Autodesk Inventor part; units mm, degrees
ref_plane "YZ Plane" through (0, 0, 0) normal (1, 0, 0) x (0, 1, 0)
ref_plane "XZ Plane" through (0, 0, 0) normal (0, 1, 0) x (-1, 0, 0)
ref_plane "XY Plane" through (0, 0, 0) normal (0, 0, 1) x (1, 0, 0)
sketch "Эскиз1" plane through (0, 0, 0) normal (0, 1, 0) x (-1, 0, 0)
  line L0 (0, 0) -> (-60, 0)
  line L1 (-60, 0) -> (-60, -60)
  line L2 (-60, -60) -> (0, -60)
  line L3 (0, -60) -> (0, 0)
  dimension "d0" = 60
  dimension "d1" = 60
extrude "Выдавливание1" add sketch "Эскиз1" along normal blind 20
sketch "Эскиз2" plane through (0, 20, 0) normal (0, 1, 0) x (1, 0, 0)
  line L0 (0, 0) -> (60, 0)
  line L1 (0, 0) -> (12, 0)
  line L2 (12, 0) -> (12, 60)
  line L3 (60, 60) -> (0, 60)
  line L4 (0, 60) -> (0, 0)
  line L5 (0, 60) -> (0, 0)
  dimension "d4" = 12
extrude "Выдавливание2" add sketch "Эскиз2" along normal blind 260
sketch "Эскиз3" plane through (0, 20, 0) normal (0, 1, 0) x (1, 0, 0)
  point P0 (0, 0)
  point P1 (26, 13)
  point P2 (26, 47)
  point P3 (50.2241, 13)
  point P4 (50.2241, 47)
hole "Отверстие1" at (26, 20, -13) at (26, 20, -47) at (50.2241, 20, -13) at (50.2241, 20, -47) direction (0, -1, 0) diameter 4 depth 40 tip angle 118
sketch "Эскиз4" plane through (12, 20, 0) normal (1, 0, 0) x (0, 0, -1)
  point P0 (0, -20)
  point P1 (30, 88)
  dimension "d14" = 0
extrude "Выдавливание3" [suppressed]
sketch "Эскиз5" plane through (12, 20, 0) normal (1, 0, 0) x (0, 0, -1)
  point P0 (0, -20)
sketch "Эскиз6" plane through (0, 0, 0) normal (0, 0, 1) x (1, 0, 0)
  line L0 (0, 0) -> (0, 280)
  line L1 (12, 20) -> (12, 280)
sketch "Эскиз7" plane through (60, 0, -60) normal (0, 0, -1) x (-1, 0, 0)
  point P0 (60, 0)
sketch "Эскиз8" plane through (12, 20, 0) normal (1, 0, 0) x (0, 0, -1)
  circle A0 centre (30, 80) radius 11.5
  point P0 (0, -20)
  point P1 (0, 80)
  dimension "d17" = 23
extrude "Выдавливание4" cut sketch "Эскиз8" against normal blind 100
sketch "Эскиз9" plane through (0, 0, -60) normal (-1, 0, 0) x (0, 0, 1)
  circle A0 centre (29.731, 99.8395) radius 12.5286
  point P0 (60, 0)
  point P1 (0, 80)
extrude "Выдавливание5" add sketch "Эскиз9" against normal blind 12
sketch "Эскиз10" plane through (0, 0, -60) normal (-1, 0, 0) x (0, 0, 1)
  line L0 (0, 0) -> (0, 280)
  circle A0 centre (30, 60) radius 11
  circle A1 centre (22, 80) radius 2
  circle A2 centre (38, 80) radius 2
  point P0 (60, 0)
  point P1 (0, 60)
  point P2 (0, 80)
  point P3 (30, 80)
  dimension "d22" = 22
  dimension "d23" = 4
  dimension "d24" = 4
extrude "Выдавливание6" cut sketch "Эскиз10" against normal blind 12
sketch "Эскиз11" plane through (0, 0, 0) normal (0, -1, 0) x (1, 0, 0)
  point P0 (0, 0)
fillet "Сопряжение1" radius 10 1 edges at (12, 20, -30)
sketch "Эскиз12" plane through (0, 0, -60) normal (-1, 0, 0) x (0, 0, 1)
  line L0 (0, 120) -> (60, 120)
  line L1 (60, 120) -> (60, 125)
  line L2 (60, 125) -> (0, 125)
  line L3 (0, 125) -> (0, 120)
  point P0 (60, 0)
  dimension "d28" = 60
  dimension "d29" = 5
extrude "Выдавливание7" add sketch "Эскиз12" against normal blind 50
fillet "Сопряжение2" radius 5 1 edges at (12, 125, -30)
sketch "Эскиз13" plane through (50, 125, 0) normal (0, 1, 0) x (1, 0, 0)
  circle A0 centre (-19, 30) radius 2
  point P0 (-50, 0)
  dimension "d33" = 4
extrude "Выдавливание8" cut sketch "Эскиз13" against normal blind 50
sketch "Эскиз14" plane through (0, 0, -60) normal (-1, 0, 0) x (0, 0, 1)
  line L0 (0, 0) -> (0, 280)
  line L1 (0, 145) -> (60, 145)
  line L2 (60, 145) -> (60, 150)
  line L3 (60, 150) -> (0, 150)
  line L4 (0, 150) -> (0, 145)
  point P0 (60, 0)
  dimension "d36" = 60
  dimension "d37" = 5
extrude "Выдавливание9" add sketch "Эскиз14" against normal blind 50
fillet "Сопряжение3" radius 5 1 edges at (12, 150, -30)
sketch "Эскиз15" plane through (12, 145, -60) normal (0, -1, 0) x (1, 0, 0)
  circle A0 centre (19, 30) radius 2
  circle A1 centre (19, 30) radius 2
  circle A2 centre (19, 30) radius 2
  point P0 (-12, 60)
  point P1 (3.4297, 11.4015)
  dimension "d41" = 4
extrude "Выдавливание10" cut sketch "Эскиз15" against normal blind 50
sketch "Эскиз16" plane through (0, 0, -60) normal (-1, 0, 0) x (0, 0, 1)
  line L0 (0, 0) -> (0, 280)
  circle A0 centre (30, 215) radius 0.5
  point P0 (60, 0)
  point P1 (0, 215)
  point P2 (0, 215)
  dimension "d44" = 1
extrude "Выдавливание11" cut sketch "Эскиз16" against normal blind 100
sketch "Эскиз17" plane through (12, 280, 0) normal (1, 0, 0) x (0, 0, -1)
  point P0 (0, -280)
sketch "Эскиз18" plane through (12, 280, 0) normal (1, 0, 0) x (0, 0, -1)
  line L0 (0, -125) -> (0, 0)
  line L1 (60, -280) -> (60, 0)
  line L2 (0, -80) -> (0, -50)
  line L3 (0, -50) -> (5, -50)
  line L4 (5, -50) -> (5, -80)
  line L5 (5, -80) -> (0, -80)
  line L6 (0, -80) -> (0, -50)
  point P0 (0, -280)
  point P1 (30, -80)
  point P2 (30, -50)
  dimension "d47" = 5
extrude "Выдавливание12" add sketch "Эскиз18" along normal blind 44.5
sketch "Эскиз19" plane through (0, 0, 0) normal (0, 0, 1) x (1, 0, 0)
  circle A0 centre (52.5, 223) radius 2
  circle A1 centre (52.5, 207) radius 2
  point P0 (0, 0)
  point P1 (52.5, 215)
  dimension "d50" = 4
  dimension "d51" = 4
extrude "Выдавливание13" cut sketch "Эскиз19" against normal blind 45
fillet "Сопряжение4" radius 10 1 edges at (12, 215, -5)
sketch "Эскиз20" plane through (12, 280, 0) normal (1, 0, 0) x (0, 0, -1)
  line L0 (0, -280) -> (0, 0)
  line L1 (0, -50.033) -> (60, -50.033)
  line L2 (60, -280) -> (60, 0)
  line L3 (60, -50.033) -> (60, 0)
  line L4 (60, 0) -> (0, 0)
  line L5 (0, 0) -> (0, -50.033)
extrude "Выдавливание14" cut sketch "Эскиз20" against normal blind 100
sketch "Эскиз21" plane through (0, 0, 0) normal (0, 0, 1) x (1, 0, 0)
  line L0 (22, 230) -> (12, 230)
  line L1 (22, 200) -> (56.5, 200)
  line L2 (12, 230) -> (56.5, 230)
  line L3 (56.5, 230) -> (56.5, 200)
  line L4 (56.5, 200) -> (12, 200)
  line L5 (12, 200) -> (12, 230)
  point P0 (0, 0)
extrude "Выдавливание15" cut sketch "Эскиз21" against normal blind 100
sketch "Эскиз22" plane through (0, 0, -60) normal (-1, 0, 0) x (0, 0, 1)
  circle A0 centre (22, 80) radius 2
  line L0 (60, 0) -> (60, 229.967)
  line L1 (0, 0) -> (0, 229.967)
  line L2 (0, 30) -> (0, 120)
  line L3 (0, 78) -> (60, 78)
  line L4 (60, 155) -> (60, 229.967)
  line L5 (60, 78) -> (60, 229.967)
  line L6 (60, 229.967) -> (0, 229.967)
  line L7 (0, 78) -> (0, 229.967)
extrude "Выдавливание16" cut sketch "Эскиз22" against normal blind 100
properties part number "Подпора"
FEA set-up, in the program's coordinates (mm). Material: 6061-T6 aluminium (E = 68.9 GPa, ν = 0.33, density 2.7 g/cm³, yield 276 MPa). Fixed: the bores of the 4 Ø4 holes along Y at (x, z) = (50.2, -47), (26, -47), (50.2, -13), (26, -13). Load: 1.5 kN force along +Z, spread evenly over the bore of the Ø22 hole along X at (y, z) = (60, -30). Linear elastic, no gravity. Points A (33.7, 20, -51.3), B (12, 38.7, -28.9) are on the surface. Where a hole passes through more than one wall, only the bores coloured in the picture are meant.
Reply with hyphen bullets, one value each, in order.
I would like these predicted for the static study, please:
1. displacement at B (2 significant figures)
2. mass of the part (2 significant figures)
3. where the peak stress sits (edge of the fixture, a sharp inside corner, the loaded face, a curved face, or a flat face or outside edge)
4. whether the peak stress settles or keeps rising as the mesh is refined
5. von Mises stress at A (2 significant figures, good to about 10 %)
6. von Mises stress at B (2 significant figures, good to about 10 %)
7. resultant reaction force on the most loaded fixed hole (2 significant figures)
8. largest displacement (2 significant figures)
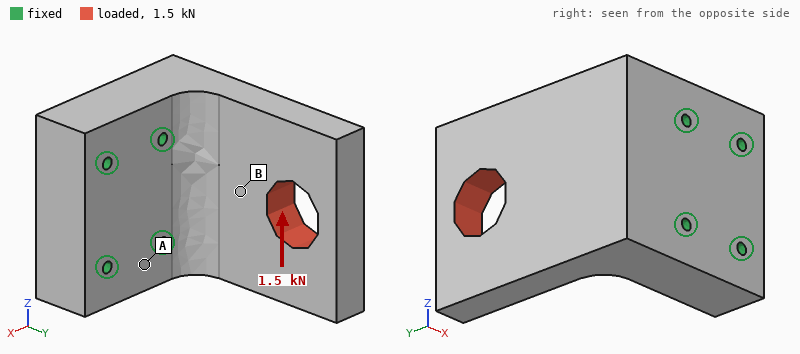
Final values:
- 11 µm
- 300 g
- edge of the fixture
- keeps rising
- 3.2 MPa
- 9.1 MPa
- 1.9 kN
- 31 µm
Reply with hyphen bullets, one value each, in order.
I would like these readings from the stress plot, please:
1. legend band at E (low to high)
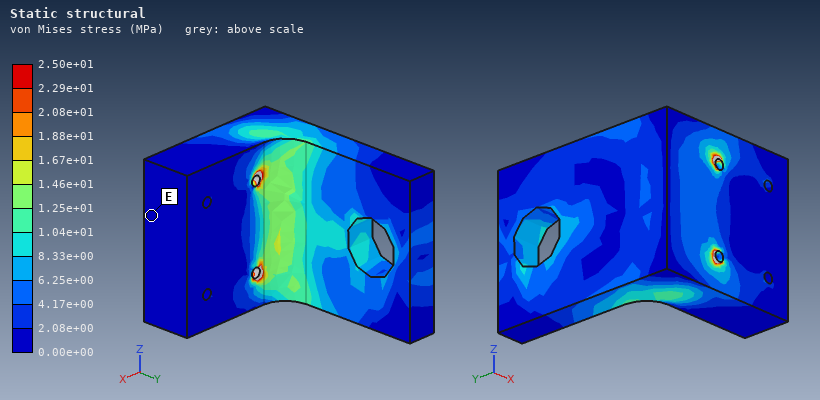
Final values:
- 0.00e+00 to 2.08e+00 MPa
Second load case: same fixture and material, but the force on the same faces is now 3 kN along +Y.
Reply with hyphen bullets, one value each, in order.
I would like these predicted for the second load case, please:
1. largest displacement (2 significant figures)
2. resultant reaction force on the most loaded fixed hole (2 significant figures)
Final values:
- 30 µm
- 1.8 kN
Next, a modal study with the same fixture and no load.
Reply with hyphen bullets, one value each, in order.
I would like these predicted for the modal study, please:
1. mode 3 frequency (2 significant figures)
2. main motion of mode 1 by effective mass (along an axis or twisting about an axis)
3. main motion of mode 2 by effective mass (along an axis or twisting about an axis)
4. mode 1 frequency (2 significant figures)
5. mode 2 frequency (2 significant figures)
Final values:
- 5700 Hz
- along X
- along Z
- 2600 Hz
- 4700 Hz
